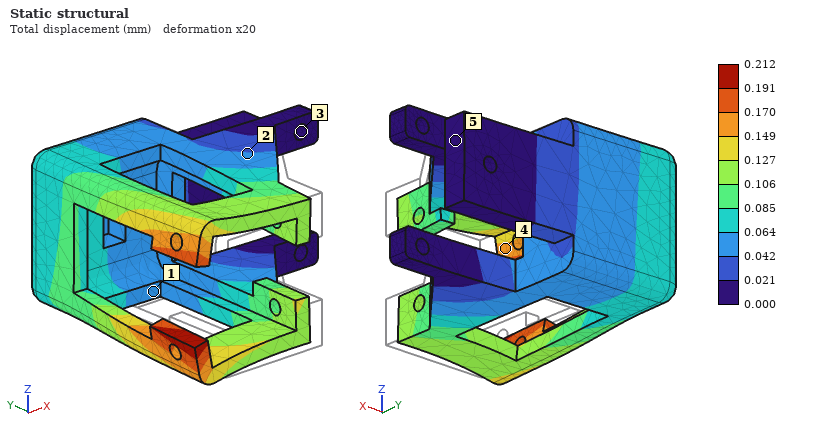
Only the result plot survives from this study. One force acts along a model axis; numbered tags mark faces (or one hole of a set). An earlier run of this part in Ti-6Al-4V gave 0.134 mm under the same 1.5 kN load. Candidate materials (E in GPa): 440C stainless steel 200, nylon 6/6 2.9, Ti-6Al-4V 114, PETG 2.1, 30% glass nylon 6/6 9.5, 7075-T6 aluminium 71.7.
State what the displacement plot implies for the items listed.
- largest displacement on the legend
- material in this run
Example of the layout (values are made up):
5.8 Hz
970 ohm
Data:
0.212 mm
7075-T6 aluminium
